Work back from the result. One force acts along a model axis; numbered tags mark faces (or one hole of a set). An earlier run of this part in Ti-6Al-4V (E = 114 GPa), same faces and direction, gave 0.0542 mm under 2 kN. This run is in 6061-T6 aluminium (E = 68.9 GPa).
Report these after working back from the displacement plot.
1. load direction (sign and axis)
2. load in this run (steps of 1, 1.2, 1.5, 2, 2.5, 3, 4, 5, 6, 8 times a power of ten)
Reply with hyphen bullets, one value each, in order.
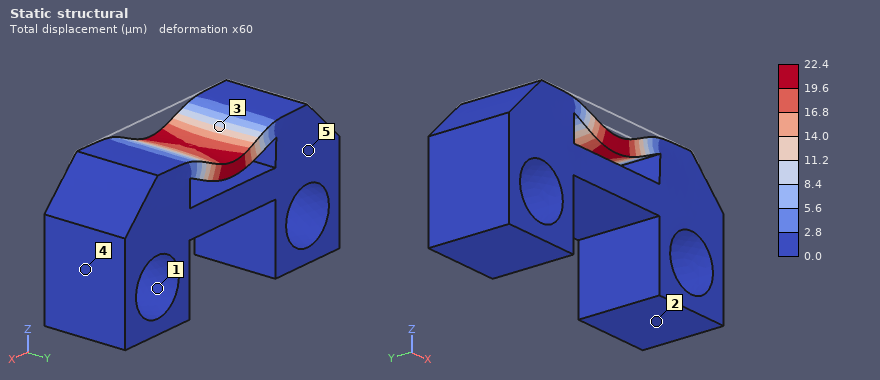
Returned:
- -Z
- 500 N
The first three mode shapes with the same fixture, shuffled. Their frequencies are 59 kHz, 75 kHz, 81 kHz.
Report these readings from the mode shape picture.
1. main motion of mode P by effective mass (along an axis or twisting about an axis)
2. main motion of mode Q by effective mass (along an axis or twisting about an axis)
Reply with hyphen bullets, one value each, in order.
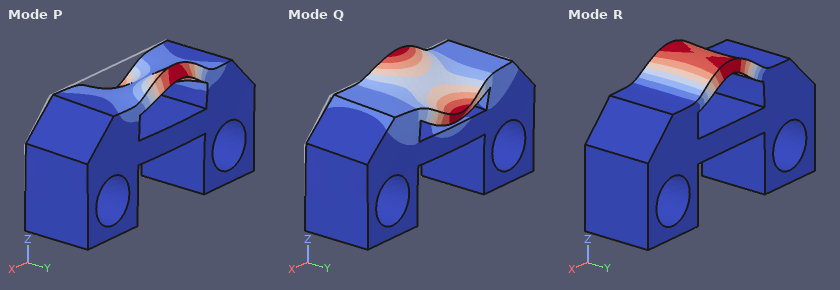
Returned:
- along Y
- along Y
